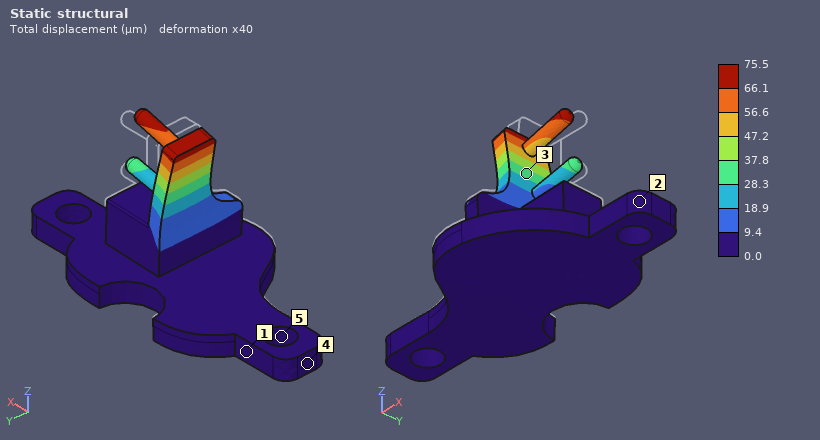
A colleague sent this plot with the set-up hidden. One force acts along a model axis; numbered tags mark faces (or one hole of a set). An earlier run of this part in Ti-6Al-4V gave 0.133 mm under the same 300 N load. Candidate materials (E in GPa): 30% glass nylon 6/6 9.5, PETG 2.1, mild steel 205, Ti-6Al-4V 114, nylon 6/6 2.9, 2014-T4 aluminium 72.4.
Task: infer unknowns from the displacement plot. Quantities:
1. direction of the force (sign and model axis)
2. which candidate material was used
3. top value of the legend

-X
mild steel
75.5 µm
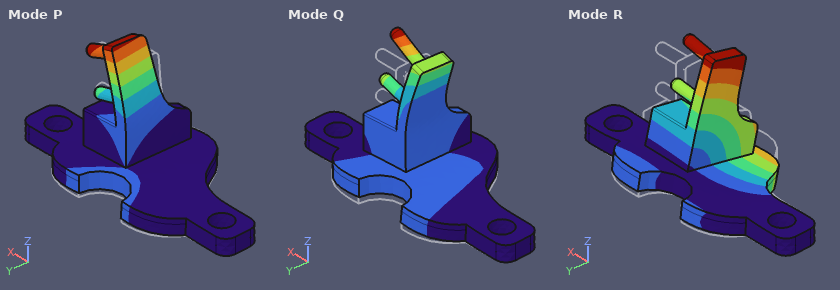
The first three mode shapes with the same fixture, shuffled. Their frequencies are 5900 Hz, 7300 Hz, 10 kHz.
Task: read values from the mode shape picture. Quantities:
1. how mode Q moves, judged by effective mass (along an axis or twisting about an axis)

along Z
